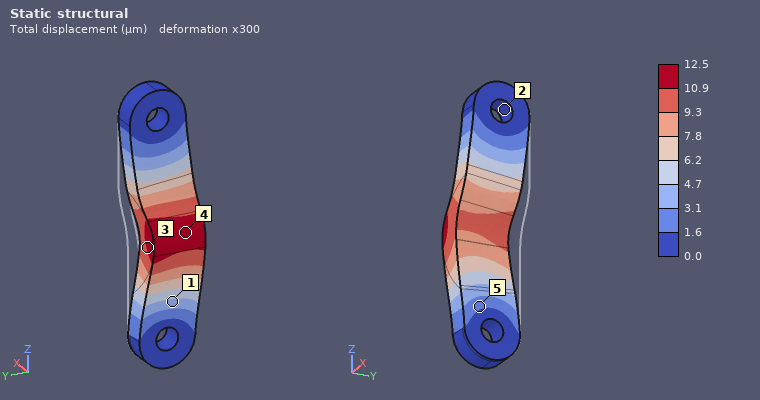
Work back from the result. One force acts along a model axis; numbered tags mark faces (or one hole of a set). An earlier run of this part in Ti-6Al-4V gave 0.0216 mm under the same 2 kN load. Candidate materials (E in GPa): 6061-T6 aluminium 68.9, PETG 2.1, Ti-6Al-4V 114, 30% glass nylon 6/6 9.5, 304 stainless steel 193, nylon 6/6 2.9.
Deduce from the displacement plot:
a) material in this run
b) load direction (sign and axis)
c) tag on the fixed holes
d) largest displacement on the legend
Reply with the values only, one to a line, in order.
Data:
304 stainless steel
-Y
2
12.5 µm
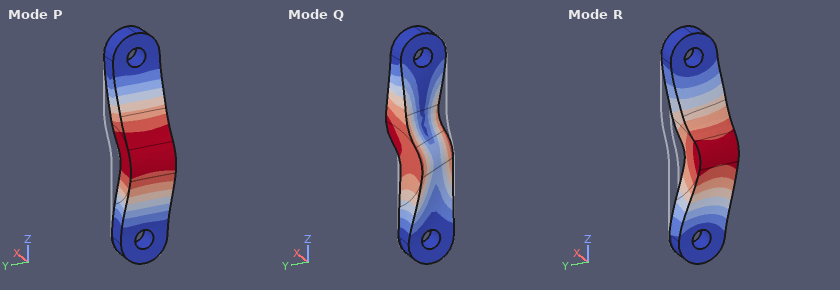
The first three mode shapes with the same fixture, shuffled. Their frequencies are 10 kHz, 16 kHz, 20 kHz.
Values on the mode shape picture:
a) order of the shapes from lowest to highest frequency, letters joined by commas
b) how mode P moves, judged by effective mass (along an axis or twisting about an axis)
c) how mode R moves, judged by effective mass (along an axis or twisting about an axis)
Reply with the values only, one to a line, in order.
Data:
P, R, Q
along X
along Y
